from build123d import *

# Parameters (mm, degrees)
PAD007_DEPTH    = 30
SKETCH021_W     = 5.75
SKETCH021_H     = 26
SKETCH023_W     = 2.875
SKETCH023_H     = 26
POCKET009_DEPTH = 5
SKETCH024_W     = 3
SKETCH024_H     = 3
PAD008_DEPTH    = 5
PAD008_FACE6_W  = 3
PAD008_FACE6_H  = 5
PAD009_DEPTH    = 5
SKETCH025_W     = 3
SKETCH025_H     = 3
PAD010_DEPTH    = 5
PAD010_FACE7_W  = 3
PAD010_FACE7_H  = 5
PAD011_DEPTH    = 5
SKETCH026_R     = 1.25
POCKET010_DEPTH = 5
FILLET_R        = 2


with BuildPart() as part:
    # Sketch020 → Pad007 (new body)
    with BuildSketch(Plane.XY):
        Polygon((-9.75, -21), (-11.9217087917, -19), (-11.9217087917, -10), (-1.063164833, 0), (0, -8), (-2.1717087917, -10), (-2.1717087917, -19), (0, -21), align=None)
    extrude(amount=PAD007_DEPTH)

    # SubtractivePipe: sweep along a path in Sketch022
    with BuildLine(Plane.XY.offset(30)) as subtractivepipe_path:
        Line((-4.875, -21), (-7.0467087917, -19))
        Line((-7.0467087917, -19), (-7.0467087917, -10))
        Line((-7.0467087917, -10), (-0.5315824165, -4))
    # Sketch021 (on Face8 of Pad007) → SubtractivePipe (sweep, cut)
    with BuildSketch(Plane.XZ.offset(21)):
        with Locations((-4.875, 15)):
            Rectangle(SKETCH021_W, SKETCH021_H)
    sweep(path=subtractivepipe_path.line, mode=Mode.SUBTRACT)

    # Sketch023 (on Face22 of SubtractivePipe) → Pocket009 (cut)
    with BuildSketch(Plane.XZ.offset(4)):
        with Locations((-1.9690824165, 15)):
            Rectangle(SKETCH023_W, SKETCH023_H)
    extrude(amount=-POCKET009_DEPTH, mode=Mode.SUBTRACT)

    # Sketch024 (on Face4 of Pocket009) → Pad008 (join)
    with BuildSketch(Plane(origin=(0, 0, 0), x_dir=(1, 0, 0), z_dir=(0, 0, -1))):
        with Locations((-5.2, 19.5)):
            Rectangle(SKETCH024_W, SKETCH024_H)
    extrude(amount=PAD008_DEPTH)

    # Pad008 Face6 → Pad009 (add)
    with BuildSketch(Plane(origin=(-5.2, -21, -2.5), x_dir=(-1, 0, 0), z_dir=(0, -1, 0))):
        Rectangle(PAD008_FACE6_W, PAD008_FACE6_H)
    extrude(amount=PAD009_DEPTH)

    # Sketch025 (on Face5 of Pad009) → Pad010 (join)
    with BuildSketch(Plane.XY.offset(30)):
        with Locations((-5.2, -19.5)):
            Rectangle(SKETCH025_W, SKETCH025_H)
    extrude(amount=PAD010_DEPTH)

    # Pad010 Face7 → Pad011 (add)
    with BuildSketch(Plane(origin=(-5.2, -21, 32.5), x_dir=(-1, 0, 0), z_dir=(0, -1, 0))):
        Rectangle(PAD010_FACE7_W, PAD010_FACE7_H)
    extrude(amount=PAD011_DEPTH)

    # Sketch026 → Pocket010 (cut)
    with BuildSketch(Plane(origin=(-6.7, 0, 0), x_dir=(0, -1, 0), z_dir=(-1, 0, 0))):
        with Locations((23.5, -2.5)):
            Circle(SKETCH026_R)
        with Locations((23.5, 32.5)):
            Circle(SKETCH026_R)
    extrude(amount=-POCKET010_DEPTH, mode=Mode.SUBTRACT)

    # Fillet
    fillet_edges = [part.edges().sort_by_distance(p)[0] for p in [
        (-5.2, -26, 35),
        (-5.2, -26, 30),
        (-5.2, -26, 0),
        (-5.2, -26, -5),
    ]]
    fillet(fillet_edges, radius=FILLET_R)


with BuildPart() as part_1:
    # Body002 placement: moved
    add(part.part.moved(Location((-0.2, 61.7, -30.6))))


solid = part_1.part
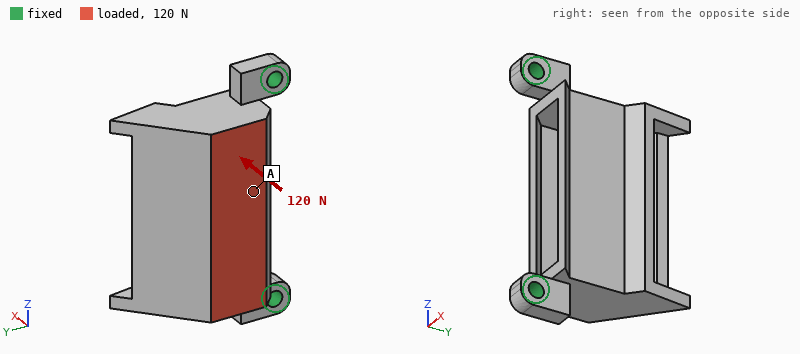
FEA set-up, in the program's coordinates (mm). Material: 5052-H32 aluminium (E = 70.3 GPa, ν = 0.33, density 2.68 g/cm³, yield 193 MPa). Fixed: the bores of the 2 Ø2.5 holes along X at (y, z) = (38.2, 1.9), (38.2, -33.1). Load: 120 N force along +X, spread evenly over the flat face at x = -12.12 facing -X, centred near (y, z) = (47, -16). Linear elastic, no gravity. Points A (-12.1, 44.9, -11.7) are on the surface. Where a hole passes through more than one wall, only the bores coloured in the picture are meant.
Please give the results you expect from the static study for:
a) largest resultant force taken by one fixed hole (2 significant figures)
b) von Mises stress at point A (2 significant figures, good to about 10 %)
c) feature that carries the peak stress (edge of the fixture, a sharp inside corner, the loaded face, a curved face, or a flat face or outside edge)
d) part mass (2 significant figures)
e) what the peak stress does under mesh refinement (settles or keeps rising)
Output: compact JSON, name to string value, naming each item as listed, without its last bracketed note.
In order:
{"largest resultant force taken by one fixed hole": "61 N", "von Mises stress at point A": "8.8 MPa", "feature that carries the peak stress": "edge of the fixture", "part mass": "6.7 g", "what the peak stress does under mesh refinement": "keeps rising"}
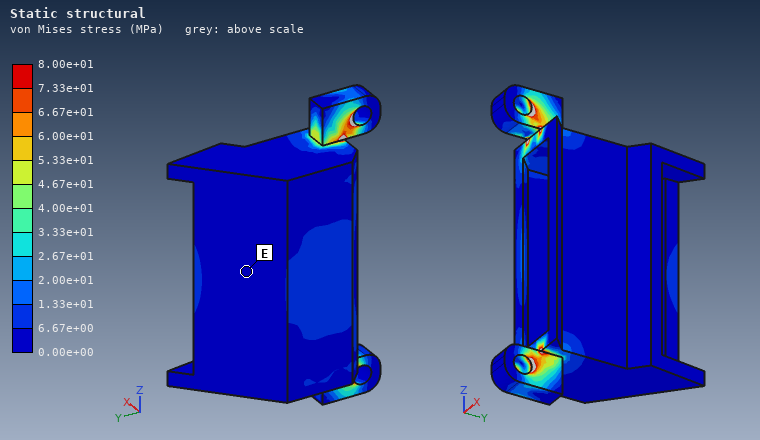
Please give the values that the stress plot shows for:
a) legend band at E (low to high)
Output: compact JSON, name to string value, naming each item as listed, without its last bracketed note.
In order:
{"legend band at E": "0.00e+00 to 6.67e+00 MPa"}
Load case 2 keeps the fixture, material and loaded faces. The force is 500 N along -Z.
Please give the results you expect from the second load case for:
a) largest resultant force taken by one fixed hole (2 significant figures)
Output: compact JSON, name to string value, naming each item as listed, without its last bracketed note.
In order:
{"largest resultant force taken by one fixed hole": "280 N"}
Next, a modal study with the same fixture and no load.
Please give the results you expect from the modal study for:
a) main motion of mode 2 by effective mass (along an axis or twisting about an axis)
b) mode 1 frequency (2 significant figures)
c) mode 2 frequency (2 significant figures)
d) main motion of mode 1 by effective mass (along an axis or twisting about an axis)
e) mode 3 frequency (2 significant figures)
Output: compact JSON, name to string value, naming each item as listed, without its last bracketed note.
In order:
{"main motion of mode 2 by effective mass": "twisting about Y", "mode 1 frequency": "3000 Hz", "mode 2 frequency": "9400 Hz", "main motion of mode 1 by effective mass": "along X", "mode 3 frequency": "13 kHz"}
